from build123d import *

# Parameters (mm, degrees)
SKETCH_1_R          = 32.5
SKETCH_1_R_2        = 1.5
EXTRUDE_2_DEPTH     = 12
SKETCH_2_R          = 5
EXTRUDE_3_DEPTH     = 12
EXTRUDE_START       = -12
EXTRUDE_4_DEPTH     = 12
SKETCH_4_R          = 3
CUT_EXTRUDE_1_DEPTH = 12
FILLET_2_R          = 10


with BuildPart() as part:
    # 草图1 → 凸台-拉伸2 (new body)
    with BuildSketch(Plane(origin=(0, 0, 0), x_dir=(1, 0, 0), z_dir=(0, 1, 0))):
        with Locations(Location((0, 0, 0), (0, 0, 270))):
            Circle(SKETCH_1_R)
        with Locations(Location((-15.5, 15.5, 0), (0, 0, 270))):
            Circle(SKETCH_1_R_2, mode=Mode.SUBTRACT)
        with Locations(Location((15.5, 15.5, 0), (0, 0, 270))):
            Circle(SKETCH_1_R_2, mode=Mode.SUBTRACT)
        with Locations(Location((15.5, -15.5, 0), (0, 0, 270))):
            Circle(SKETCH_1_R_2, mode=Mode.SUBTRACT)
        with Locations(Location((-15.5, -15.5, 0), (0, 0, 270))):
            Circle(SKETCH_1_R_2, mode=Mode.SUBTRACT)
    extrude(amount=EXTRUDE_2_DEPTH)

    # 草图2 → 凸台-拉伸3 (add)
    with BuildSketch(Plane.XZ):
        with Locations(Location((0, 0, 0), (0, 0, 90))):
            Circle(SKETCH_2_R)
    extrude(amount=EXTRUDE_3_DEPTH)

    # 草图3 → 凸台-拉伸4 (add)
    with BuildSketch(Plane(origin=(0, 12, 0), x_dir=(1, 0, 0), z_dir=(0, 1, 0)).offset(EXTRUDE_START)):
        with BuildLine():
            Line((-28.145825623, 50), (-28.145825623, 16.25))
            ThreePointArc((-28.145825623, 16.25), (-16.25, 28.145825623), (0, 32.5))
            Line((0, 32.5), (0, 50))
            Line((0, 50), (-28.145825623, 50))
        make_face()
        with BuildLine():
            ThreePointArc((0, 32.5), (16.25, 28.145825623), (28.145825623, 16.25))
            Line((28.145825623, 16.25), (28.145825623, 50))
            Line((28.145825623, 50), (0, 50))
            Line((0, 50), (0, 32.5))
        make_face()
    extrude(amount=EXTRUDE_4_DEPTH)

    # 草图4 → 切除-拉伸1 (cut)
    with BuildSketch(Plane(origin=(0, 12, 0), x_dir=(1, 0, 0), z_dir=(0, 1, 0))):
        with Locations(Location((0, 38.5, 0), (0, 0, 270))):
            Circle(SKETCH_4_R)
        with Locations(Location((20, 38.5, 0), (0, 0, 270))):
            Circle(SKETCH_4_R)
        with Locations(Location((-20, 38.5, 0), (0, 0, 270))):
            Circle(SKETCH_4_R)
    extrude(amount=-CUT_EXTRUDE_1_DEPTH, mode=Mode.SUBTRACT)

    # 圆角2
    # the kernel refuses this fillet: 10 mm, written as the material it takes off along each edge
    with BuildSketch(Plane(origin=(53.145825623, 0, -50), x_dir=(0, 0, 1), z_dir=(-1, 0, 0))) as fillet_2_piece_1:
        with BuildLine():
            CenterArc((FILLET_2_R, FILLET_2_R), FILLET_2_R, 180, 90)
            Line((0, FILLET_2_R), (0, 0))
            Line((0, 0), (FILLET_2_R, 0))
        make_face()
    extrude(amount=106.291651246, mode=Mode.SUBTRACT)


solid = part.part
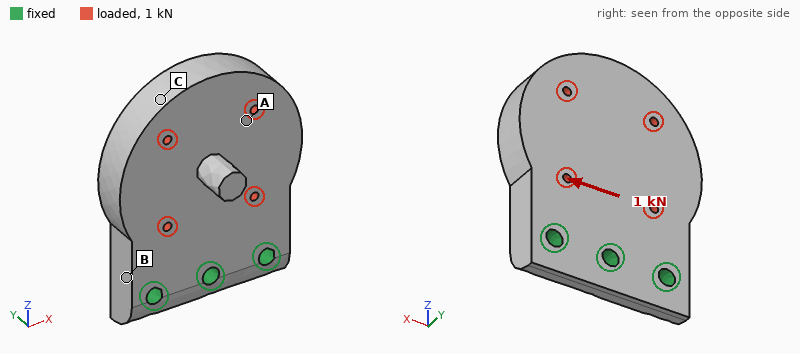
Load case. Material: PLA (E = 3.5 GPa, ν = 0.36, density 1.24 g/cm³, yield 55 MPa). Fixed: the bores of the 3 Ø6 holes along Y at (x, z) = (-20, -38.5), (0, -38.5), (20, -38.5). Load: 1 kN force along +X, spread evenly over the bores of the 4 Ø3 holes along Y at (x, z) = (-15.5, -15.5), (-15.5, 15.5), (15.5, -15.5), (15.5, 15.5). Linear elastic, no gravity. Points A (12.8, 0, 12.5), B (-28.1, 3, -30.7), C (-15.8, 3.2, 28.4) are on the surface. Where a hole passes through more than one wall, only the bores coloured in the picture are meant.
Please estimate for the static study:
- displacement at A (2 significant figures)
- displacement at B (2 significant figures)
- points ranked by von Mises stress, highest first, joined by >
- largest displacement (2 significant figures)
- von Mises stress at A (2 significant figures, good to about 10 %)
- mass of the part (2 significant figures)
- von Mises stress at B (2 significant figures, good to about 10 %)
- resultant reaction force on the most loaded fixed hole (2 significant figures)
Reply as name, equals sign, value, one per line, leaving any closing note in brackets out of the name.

displacement at A = 0.10 mm
displacement at B = 0.026 mm
points ranked by von Mises stress, highest first, joined by > = B > A > C
largest displacement = 0.13 mm
von Mises stress at A = 1.8 MPa
mass of the part = 66 g
von Mises stress at B = 4.1 MPa
resultant reaction force on the most loaded fixed hole = 930 N
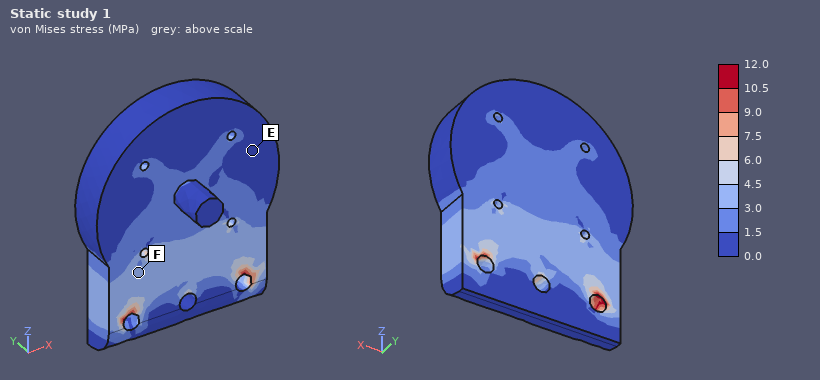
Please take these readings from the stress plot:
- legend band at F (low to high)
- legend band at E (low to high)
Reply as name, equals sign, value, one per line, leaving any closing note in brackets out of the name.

legend band at F = 3.0 to 4.5 MPa
legend band at E = 0.0 to 1.5 MPa
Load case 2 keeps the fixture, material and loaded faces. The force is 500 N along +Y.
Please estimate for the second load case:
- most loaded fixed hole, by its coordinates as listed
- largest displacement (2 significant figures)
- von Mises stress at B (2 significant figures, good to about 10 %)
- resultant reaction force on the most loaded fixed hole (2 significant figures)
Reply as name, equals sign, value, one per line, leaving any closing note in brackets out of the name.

most loaded fixed hole, by its coordinates as listed = (0, -38.5)
largest displacement = 0.80 mm
von Mises stress at B = 4.1 MPa
resultant reaction force on the most loaded fixed hole = 240 N
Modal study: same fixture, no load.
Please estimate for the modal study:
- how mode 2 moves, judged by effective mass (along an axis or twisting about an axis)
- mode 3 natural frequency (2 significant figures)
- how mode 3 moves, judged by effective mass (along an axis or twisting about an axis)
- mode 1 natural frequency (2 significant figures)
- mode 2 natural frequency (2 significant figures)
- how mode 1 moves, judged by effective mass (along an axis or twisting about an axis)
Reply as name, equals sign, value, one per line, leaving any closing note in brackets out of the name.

how mode 2 moves, judged by effective mass = twisting about Z
mode 3 natural frequency = 2300 Hz
how mode 3 moves, judged by effective mass = along X
mode 1 natural frequency = 720 Hz
mode 2 natural frequency = 1800 Hz
how mode 1 moves, judged by effective mass = along Y
